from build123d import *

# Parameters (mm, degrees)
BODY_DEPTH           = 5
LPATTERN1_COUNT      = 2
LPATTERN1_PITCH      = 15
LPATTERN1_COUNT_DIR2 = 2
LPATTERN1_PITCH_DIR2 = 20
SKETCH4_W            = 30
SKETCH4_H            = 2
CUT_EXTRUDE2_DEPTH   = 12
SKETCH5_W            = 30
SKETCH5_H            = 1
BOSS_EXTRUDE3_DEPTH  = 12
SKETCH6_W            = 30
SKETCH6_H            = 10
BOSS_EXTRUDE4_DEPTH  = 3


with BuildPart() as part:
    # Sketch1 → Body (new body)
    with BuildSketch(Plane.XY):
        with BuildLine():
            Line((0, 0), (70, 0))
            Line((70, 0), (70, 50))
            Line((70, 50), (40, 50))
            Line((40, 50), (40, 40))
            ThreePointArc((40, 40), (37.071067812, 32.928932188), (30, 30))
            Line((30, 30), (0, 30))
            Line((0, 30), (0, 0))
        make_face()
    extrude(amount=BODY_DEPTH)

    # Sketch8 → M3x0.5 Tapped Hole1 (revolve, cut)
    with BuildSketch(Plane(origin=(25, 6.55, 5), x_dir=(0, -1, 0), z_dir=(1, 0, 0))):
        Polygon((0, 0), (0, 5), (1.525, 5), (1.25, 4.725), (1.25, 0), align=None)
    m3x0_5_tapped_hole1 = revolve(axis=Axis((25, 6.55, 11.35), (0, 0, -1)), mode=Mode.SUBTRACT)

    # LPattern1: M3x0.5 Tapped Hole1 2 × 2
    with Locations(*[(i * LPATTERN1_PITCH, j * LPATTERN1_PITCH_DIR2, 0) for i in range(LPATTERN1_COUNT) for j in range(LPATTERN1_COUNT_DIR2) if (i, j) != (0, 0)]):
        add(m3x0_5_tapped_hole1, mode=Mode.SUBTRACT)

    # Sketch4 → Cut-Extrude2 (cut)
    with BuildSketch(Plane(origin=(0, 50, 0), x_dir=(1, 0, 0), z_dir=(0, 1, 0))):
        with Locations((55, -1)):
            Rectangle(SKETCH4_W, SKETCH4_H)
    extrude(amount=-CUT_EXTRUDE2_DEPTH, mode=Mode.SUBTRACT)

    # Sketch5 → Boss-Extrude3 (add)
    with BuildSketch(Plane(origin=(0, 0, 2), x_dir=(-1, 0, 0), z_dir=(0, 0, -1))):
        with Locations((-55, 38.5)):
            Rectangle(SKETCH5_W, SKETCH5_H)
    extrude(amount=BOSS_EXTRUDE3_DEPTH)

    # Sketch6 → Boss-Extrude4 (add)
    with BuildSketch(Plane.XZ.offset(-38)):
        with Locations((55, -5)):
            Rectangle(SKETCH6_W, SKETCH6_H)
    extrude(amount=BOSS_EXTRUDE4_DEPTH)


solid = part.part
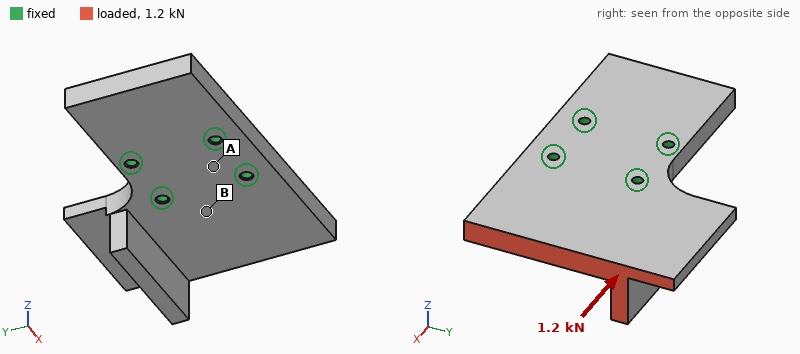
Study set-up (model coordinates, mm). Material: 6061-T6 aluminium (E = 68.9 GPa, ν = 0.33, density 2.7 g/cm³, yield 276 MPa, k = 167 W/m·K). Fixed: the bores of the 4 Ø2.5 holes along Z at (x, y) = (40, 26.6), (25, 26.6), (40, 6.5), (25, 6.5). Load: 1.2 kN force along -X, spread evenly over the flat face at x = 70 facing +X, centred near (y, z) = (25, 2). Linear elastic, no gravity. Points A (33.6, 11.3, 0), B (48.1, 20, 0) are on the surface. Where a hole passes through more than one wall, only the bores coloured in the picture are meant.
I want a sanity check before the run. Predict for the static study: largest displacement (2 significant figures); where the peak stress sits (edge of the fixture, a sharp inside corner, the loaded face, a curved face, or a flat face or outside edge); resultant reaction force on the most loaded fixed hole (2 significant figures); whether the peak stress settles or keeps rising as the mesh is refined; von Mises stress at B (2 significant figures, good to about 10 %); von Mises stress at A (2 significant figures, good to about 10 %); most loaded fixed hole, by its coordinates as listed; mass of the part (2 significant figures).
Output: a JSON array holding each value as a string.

["25 µm", "edge of the fixture", "840 N", "keeps rising", "10 MPa", "2.7 MPa", "(40, 26.6)", "38 g"]
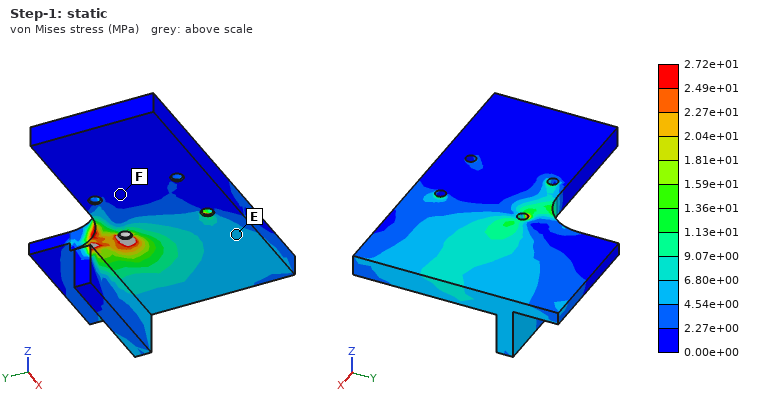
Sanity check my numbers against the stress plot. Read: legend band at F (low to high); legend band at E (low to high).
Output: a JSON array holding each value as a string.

["0.00e+00 to 2.27e+00 MPa", "4.54e+00 to 6.80e+00 MPa"]
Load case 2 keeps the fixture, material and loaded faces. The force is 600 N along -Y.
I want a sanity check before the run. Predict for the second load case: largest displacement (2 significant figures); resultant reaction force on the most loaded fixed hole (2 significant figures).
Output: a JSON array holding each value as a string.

["27 µm", "740 N"]
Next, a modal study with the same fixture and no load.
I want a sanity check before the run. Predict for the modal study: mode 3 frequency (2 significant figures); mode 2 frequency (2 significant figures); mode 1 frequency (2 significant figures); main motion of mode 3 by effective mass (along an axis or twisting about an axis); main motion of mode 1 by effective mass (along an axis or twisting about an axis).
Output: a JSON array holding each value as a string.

["5900 Hz", "5400 Hz", "3200 Hz", "along Z", "along Z"]
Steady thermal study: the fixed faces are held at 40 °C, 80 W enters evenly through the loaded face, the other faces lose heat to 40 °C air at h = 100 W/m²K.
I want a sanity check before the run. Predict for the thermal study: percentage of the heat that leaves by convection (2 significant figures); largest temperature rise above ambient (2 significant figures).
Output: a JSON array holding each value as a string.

["19 %", "64 K"]
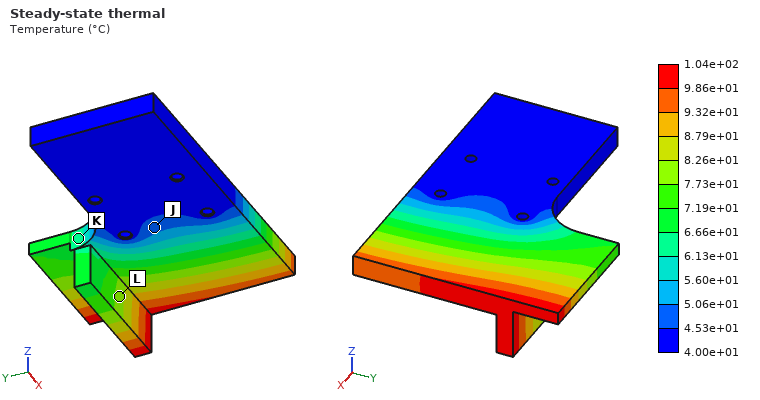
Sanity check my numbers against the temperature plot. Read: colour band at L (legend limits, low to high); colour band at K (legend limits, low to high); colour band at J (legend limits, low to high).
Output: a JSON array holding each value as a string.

["7.73e+01 to 8.26e+01 °C", "6.13e+01 to 6.66e+01 °C", "4.53e+01 to 5.06e+01 °C"]
